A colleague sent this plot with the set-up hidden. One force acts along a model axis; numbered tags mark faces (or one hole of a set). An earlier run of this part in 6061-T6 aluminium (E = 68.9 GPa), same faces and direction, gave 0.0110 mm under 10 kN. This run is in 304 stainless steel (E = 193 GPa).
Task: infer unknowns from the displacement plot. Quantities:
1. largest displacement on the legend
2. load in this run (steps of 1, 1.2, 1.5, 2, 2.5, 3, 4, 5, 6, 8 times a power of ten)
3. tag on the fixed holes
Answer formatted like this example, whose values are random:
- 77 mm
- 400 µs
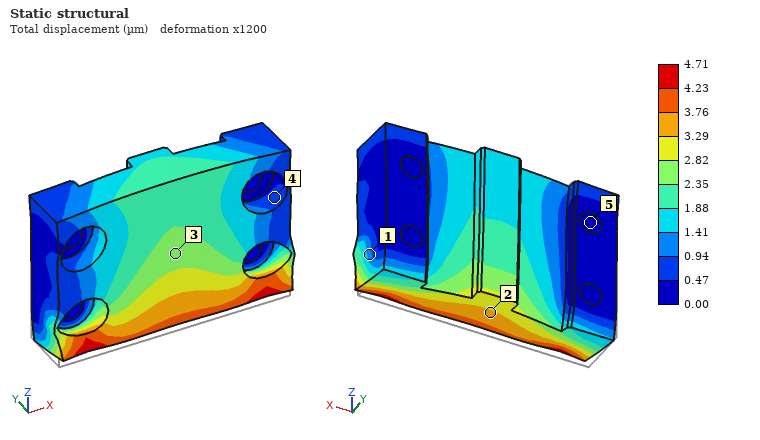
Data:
- 4.71 µm
- 12 kN
- 5
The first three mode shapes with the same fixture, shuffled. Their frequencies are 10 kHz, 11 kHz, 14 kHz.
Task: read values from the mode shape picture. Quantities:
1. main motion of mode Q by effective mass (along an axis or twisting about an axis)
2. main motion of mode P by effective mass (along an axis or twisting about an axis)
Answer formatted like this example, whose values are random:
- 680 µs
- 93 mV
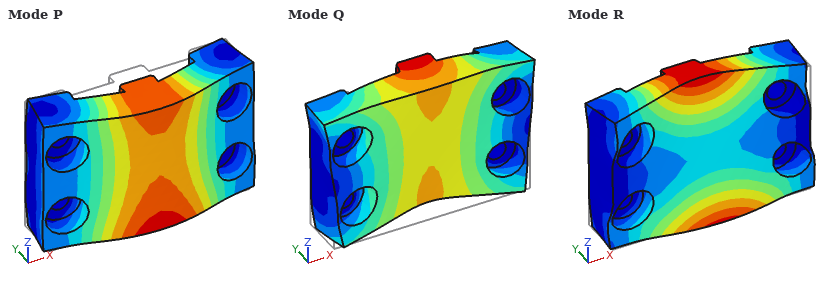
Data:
- along Z
- along Y
